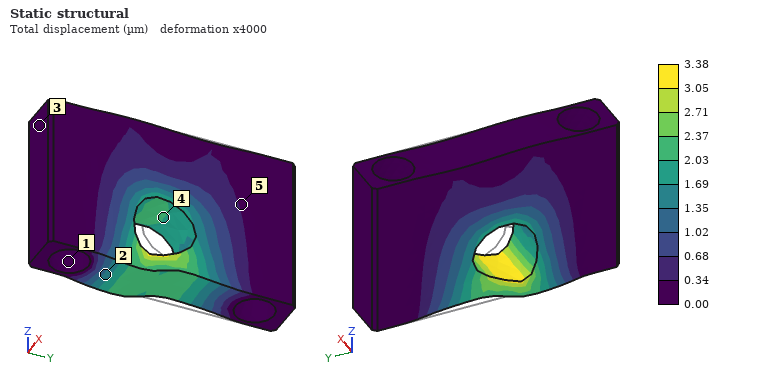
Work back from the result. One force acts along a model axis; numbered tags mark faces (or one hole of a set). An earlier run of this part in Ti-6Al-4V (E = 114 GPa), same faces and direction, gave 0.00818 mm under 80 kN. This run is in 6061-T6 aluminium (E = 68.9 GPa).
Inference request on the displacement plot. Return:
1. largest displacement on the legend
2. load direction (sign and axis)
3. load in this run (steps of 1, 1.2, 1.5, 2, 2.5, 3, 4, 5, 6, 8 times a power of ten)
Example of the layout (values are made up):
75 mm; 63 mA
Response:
3.38 µm; -Y; 20 kN
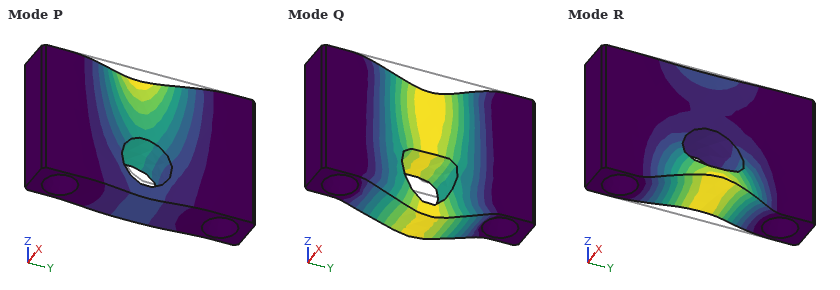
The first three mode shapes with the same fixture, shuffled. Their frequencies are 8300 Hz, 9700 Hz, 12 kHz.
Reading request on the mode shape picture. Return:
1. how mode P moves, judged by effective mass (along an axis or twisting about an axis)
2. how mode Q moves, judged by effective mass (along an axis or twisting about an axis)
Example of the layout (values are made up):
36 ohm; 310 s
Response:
along X; along Z
